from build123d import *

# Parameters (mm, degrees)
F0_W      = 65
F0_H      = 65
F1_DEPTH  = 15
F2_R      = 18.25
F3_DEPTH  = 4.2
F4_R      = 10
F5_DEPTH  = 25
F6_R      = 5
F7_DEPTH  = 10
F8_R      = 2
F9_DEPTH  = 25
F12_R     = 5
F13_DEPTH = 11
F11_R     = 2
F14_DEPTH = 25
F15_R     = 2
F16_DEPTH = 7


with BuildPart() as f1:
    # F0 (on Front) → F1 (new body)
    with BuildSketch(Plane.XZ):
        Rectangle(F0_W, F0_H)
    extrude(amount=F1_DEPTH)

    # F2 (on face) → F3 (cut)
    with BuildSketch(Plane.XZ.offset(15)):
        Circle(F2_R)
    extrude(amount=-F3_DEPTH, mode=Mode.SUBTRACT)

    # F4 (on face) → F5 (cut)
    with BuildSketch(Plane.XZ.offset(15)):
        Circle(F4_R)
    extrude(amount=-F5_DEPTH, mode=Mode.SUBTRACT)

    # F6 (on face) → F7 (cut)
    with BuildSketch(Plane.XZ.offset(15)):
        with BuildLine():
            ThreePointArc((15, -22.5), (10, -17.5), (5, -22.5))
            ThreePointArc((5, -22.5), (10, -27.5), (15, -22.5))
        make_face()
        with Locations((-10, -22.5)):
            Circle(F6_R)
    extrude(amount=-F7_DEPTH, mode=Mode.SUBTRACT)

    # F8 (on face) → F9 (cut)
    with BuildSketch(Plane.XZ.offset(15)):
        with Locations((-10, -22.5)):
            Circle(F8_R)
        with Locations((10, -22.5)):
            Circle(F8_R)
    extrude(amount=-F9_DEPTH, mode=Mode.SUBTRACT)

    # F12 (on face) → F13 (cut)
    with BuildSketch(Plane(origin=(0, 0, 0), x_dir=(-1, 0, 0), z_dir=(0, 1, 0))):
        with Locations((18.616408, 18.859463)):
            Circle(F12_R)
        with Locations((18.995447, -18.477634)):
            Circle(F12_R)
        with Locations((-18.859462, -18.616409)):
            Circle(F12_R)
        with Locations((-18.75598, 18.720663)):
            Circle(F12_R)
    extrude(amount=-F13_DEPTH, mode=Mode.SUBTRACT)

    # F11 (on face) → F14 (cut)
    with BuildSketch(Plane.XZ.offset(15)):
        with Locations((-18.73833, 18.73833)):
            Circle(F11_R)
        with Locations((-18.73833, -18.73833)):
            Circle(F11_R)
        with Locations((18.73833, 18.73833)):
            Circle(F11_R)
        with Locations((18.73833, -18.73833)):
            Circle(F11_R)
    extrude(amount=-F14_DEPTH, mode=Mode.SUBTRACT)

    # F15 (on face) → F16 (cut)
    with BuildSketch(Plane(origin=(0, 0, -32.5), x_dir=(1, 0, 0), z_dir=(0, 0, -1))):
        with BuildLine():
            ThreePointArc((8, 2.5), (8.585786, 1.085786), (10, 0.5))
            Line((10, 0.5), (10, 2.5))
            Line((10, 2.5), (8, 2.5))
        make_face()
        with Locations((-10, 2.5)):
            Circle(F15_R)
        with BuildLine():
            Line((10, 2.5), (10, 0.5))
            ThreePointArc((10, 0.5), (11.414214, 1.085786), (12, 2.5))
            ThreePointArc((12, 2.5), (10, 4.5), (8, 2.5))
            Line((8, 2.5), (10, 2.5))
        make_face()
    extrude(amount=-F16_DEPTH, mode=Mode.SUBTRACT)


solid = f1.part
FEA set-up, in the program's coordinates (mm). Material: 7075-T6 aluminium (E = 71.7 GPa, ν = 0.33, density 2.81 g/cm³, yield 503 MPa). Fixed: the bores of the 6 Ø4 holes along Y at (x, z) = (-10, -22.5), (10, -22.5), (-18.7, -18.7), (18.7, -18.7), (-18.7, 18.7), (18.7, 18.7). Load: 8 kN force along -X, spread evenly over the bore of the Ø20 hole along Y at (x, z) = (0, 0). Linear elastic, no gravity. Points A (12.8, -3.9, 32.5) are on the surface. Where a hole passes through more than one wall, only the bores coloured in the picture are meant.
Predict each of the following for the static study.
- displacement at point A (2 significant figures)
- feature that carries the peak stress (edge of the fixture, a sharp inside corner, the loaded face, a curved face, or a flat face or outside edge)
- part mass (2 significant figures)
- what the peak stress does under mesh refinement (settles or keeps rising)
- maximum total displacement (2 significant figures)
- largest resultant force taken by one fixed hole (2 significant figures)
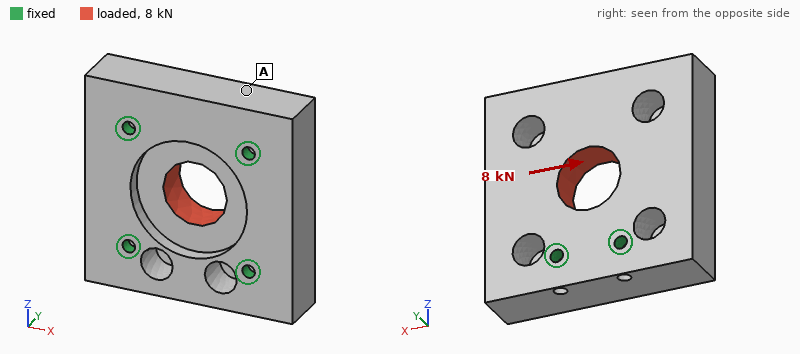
4.2 µm
edge of the fixture
140 g
keeps rising
9.5 µm
2.0 kN
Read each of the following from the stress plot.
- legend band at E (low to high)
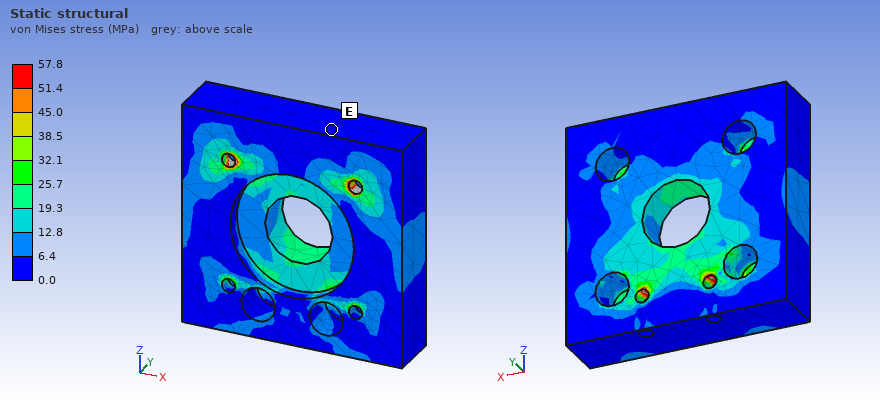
0.0 to 6.4 MPa
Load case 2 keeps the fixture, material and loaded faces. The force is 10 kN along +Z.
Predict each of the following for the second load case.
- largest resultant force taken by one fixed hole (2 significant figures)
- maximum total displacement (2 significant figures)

2.0 kN
12 µm
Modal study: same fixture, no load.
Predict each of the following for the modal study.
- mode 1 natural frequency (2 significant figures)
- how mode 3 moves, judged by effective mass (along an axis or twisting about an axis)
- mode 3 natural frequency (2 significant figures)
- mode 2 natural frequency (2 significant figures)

14 kHz
along Y
15 kHz
14 kHz
